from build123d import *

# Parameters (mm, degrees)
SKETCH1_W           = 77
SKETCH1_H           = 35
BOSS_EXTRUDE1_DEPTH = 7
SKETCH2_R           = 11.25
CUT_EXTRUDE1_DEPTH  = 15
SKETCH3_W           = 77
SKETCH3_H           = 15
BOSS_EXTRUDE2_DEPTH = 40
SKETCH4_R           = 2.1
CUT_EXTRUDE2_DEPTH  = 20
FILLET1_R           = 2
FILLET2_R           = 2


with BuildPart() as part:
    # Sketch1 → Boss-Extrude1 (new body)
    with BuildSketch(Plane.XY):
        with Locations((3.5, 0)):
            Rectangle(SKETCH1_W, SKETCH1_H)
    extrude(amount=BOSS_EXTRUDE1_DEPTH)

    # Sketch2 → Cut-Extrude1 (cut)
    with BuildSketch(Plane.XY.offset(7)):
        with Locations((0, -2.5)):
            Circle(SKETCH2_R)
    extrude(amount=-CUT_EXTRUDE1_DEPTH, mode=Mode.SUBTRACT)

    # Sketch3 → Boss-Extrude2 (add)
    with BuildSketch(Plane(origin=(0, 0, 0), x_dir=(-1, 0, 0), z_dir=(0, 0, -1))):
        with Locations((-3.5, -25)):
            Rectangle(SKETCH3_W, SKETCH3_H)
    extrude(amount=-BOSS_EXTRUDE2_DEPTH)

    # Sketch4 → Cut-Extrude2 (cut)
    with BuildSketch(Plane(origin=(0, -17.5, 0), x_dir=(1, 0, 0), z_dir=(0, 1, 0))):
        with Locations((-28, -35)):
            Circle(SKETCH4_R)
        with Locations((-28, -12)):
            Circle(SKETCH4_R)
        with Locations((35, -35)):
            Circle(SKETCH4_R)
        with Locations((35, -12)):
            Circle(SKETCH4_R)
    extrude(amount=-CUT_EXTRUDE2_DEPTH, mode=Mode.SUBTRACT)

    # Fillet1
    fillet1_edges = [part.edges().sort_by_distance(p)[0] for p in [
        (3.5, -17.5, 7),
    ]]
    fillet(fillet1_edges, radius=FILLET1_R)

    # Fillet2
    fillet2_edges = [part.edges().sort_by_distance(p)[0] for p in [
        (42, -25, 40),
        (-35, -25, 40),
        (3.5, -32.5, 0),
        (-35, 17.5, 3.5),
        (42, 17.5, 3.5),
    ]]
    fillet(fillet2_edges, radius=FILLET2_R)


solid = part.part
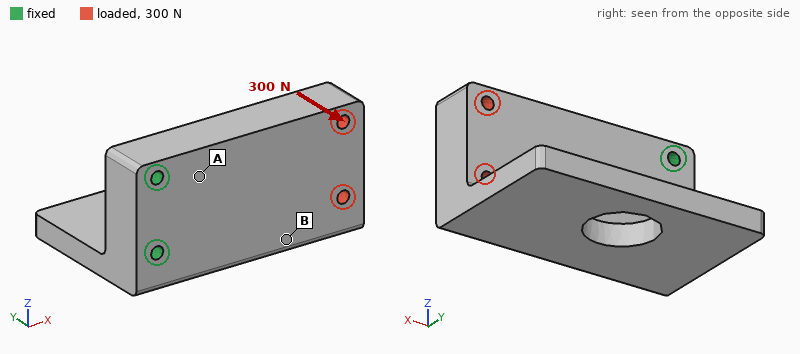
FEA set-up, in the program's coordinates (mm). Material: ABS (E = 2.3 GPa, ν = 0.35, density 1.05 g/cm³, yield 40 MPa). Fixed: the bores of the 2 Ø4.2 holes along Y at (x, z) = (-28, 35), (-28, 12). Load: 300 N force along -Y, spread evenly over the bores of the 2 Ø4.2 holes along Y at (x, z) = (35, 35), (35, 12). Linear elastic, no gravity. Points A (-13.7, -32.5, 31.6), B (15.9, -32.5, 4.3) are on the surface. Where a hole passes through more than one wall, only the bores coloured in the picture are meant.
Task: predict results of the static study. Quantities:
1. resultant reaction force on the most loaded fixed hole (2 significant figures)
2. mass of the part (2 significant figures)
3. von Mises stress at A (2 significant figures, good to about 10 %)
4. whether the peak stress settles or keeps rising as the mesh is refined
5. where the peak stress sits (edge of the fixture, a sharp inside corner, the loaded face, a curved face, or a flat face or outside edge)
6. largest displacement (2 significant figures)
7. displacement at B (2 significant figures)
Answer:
150 N
64 g
7.1 MPa
keeps rising
edge of the fixture
0.96 mm
0.49 mm
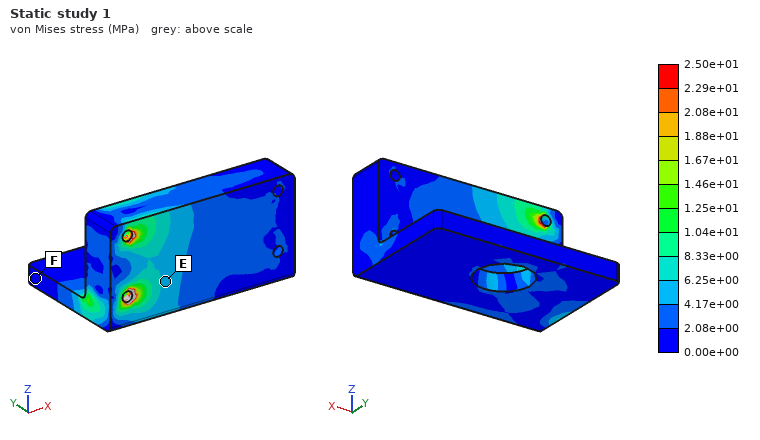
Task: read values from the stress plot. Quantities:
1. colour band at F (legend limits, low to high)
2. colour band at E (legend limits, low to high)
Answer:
0.00e+00 to 2.08e+00 MPa
4.17e+00 to 6.25e+00 MPa
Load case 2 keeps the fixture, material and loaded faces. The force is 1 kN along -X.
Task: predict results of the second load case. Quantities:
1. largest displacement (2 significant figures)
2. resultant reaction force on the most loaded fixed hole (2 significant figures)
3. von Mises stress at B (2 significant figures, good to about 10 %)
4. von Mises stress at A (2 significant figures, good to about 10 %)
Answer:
89 µm
510 N
1.1 MPa
2.2 MPa
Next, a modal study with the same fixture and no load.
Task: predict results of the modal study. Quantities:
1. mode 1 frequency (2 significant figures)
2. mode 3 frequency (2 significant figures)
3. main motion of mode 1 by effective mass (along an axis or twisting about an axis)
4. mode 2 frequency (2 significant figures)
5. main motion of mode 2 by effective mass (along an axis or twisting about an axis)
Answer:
610 Hz
1300 Hz
along Y
840 Hz
along Z
